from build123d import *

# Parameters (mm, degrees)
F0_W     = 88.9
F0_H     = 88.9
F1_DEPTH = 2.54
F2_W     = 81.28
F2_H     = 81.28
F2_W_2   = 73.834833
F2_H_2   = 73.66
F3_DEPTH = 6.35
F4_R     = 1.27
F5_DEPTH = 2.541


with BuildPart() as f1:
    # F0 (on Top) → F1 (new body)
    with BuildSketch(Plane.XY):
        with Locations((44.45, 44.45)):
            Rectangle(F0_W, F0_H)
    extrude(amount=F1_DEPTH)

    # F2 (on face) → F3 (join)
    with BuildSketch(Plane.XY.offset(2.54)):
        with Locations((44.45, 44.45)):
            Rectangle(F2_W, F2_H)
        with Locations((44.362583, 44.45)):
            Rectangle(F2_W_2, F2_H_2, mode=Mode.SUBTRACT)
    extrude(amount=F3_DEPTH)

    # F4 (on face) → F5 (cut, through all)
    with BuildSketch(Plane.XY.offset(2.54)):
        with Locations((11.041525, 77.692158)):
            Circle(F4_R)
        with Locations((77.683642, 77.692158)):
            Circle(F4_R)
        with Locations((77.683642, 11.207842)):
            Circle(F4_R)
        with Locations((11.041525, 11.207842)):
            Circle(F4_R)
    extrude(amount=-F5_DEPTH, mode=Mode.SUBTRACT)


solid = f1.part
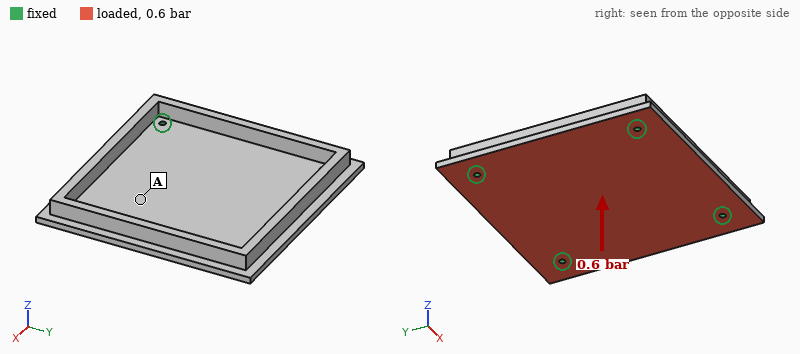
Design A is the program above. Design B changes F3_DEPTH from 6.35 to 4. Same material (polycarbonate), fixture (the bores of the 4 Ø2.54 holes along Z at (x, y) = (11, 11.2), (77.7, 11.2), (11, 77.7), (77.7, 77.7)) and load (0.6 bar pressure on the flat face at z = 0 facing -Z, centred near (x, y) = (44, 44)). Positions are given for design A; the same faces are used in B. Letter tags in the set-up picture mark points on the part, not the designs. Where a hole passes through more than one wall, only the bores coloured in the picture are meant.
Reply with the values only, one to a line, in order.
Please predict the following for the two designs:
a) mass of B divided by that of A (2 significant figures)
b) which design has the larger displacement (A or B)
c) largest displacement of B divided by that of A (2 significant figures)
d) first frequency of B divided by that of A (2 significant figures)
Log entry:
0.90
B
1.2
0.92
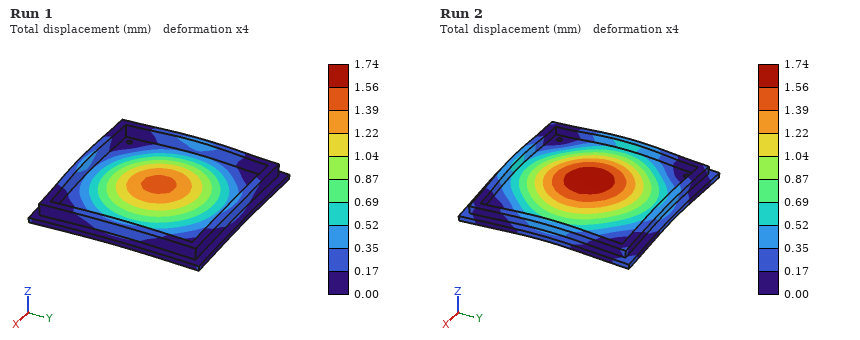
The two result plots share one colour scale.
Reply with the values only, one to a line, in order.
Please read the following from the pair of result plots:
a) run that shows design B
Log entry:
Run 2
